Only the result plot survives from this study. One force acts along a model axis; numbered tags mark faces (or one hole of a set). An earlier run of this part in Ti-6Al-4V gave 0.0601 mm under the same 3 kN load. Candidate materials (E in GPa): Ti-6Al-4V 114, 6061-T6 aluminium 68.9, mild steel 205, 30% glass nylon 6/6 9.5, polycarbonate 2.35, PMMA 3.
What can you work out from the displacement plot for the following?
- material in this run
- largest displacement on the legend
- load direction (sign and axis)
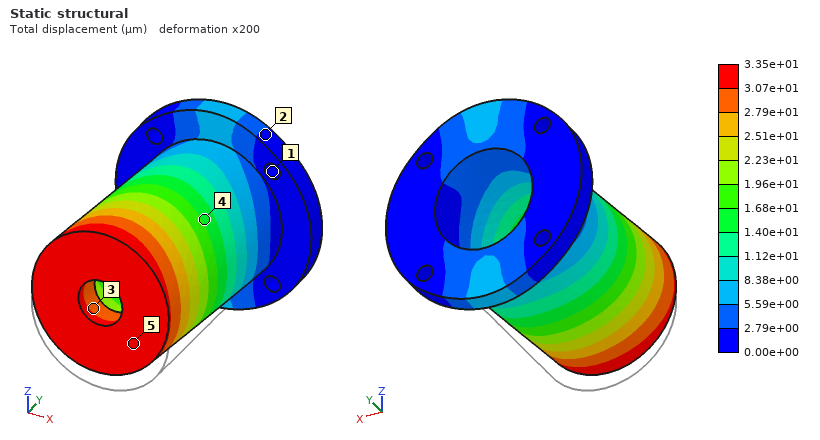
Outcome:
mild steel
3.35e+01 µm
+Z
